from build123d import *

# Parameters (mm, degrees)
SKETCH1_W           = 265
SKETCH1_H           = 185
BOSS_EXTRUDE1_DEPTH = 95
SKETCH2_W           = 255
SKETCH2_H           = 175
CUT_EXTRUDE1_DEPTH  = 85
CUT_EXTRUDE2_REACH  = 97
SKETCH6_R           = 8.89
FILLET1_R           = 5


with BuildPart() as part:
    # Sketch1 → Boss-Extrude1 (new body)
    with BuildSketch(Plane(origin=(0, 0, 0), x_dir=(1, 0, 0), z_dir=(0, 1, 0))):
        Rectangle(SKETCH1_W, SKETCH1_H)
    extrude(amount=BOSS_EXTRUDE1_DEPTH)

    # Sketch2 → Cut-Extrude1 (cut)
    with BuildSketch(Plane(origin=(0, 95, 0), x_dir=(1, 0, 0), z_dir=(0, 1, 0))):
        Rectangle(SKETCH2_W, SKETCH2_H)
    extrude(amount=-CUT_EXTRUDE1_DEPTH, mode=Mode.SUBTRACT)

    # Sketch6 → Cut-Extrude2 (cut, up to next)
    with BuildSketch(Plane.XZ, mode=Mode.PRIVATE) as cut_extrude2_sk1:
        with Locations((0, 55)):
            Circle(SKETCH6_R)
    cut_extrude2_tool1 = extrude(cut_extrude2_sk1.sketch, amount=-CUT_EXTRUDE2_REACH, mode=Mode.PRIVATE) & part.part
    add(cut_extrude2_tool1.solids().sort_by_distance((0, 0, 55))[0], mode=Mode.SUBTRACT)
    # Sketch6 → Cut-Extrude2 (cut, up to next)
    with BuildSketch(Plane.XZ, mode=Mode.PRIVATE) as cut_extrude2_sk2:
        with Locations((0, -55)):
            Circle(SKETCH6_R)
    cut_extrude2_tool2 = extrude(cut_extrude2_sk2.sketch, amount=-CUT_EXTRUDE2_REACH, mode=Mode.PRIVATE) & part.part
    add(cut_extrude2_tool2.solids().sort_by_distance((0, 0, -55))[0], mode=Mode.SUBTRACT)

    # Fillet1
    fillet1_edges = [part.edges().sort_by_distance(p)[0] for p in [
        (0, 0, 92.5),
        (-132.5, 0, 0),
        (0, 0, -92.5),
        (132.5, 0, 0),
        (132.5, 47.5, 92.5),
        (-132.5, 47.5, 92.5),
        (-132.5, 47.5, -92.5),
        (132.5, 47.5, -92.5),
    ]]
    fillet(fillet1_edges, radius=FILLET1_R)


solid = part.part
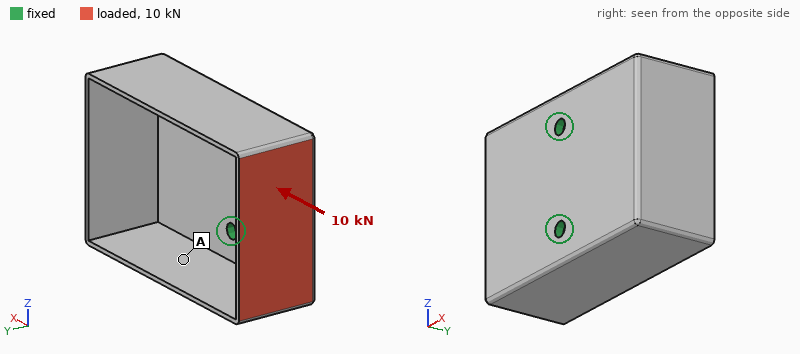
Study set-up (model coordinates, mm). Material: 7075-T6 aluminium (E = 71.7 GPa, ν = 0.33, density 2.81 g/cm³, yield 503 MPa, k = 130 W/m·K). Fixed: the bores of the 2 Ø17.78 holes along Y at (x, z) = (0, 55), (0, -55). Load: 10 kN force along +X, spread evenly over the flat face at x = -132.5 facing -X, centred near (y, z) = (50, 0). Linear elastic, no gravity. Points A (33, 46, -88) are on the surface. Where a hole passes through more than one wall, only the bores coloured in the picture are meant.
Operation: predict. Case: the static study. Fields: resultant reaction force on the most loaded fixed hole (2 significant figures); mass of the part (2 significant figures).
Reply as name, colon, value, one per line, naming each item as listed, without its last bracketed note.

resultant reaction force on the most loaded fixed hole: 5.1 kN
mass of the part: 2.4 kg
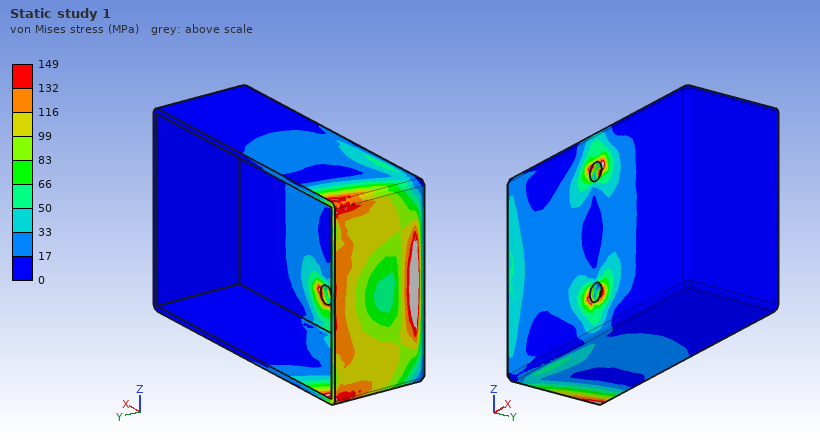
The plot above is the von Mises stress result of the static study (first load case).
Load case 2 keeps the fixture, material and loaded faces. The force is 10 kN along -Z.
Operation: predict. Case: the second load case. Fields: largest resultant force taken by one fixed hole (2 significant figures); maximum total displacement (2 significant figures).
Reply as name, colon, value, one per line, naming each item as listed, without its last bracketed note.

largest resultant force taken by one fixed hole: 12 kN
maximum total displacement: 1.3 mm
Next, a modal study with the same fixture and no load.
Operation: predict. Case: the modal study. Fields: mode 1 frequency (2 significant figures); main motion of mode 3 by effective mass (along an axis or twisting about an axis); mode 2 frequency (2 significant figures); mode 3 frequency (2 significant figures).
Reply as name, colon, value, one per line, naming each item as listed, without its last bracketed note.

mode 1 frequency: 340 Hz
main motion of mode 3 by effective mass: along Z
mode 2 frequency: 440 Hz
mode 3 frequency: 680 Hz
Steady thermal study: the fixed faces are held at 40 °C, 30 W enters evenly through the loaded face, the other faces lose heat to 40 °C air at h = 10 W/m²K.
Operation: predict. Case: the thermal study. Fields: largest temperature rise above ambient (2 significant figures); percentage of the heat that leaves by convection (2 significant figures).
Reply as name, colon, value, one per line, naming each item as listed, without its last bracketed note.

largest temperature rise above ambient: 17 K
percentage of the heat that leaves by convection: 31 %
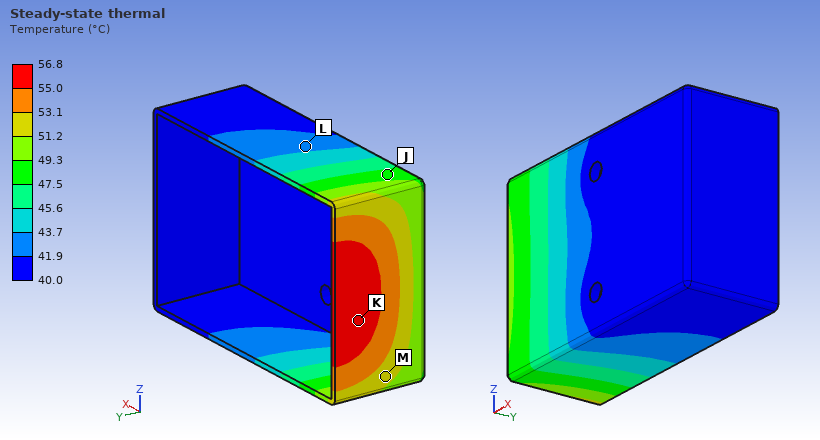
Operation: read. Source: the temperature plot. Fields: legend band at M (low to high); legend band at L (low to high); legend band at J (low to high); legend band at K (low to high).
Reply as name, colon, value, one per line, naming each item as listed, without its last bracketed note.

legend band at M: 51.2 to 53.1 °C
legend band at L: 41.9 to 43.7 °C
legend band at J: 47.5 to 49.3 °C
legend band at K: 55.0 to 56.8 °C
